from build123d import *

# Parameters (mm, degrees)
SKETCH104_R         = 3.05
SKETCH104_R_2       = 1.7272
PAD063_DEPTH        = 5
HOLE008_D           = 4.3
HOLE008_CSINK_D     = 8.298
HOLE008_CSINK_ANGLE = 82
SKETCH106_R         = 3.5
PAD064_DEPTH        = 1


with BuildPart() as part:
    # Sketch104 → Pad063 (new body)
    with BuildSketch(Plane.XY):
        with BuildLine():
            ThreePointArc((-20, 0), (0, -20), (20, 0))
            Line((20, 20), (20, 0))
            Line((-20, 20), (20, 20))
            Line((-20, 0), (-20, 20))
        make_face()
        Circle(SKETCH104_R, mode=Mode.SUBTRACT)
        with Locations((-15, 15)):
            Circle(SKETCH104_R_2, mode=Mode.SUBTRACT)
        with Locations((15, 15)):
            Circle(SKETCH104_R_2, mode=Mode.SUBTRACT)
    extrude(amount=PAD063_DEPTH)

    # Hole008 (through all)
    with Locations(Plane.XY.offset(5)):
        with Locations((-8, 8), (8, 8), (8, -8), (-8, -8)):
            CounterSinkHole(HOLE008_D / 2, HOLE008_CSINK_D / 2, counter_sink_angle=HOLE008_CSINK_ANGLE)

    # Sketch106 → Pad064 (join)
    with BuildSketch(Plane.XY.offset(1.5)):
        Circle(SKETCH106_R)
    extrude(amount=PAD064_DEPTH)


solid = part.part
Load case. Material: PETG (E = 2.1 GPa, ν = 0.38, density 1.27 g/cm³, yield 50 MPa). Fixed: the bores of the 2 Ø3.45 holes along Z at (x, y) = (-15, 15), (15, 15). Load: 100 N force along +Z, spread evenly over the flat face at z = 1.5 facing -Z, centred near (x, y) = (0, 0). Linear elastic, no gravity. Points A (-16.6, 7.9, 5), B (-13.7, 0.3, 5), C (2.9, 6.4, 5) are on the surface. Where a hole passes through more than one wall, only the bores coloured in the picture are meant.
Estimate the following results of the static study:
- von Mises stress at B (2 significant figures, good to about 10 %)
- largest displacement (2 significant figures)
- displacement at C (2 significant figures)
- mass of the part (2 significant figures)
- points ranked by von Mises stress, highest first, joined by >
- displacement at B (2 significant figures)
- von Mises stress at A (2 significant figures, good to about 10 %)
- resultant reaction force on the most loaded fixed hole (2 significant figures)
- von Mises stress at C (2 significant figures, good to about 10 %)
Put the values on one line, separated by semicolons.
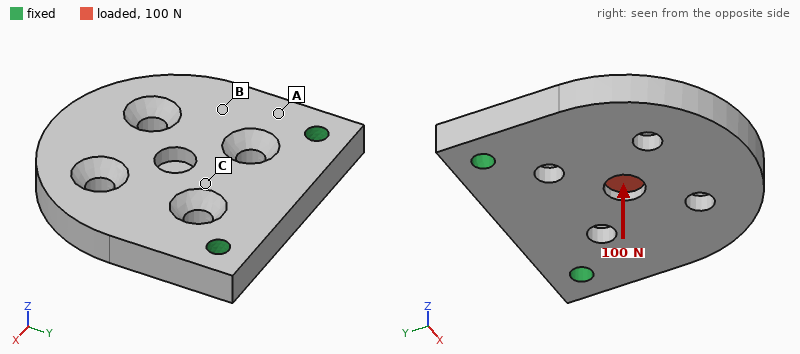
2.1 MPa; 0.67 mm; 0.16 mm; 8.2 g; A > C > B; 0.21 mm; 8.0 MPa; 50 N; 5.5 MPa
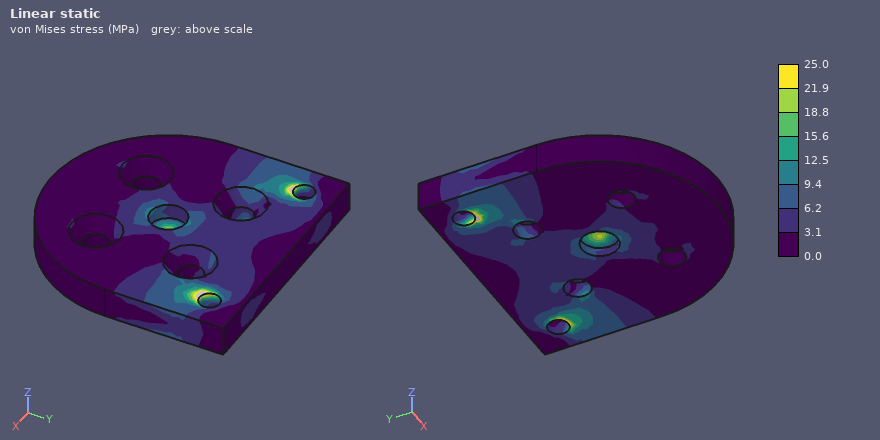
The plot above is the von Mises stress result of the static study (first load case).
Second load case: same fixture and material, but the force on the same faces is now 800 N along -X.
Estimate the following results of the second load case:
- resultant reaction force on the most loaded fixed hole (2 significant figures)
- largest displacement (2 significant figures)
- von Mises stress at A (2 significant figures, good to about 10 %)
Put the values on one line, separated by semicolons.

540 N; 0.23 mm; 8.1 MPa
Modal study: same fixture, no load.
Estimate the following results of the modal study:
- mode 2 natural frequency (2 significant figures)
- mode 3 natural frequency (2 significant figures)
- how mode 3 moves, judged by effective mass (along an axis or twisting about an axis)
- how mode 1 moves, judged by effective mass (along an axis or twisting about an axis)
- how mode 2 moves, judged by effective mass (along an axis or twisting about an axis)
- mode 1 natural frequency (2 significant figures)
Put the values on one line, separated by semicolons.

2400 Hz; 4200 Hz; along X; along Z; twisting about Y; 870 Hz
